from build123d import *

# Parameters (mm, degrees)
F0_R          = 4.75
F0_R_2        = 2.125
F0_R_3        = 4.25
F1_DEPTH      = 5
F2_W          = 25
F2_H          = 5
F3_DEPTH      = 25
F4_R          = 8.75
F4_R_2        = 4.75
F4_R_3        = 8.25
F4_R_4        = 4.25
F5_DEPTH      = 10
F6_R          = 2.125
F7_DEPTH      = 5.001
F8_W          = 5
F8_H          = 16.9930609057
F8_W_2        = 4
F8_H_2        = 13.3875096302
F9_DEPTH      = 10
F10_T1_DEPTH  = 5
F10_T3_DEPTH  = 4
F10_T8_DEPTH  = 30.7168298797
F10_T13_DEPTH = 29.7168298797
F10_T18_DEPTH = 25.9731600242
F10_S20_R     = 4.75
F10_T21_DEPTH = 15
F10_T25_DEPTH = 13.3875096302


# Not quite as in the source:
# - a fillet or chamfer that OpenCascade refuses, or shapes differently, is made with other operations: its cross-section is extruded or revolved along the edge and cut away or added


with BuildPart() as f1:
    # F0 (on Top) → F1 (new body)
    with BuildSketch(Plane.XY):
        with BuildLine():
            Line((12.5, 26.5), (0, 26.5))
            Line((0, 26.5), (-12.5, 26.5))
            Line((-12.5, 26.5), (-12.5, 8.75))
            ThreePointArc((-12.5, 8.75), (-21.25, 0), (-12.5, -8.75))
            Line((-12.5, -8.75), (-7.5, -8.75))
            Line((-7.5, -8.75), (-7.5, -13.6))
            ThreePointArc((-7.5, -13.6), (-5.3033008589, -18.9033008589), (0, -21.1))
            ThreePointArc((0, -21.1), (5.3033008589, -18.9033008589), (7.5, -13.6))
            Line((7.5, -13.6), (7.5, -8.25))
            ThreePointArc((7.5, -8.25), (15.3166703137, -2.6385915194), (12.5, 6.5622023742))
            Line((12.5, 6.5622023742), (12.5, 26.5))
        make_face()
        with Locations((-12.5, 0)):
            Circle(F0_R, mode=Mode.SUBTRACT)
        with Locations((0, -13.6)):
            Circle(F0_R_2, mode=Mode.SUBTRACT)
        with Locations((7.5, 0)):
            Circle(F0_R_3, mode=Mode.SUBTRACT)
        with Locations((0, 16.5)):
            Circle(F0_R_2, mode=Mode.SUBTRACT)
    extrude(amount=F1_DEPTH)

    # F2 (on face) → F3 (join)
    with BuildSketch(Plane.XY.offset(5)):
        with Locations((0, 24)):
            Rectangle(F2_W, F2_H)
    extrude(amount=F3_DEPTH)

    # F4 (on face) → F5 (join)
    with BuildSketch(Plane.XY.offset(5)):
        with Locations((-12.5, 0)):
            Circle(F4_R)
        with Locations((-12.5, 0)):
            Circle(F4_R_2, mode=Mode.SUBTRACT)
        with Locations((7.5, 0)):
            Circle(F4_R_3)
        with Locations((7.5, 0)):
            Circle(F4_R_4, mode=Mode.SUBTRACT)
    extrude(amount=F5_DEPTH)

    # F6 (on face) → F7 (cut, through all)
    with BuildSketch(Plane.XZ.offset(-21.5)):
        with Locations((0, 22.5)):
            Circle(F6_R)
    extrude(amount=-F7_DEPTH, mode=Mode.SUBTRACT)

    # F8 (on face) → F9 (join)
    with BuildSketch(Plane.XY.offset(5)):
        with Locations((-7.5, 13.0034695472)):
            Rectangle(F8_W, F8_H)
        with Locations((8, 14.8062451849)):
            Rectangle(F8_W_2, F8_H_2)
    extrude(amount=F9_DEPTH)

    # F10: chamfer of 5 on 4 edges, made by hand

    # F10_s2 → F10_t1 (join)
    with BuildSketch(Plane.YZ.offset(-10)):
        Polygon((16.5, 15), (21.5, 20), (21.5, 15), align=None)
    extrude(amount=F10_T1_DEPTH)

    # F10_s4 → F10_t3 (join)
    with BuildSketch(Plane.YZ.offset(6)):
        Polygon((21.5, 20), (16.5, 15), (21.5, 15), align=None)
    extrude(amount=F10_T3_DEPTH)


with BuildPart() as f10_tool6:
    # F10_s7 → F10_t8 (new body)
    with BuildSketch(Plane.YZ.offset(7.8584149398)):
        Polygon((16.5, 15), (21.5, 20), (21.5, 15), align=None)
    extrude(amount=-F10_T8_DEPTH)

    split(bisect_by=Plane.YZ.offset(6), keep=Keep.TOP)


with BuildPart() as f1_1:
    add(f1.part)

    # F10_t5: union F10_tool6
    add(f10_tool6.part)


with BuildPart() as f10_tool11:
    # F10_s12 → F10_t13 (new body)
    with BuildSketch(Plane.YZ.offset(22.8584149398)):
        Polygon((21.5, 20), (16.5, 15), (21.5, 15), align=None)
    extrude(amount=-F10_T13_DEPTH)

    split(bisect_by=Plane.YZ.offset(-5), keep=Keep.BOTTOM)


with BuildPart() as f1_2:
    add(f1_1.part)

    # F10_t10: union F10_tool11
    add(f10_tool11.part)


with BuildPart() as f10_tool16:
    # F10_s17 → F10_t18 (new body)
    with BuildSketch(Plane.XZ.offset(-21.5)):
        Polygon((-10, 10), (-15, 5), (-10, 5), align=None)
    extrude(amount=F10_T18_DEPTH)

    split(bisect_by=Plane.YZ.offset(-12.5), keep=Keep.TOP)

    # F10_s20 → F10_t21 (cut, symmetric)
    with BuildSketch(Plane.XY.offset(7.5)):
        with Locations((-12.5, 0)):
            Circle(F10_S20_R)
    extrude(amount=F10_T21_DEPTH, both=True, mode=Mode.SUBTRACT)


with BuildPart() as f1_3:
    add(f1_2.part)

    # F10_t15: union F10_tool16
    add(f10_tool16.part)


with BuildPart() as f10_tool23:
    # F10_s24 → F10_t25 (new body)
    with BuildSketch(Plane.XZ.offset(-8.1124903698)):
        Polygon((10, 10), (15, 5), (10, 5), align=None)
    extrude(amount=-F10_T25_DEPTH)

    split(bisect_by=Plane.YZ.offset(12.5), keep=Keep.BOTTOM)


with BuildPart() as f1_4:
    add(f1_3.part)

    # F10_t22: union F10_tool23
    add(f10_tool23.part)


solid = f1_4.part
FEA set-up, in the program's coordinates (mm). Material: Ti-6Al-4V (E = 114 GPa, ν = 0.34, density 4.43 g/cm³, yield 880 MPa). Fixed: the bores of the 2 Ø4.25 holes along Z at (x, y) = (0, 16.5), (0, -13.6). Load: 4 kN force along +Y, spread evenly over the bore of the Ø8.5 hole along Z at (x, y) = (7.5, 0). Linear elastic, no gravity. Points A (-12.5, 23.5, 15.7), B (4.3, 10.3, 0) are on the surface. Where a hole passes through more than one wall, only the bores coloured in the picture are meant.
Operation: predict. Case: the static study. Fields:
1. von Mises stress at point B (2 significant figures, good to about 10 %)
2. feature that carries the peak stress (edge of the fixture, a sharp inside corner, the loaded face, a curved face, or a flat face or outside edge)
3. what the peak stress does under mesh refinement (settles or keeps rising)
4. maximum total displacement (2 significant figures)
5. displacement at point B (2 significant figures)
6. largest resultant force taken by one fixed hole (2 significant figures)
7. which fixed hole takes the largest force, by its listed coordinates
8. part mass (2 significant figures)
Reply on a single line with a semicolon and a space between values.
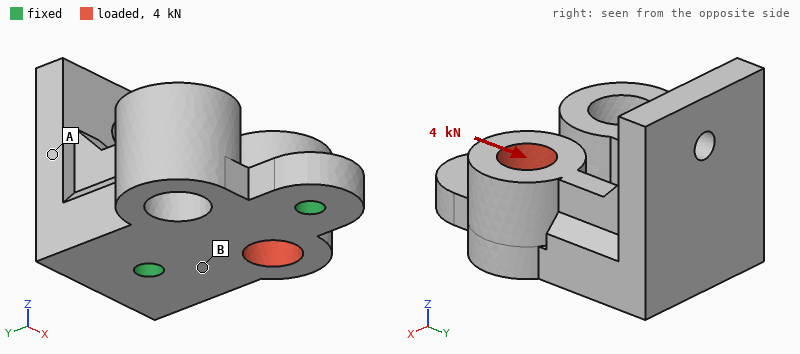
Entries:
23 MPa; edge of the fixture; keeps rising; 15 µm; 2.8 µm; 2.5 kN; (0, 16.5); 58 g
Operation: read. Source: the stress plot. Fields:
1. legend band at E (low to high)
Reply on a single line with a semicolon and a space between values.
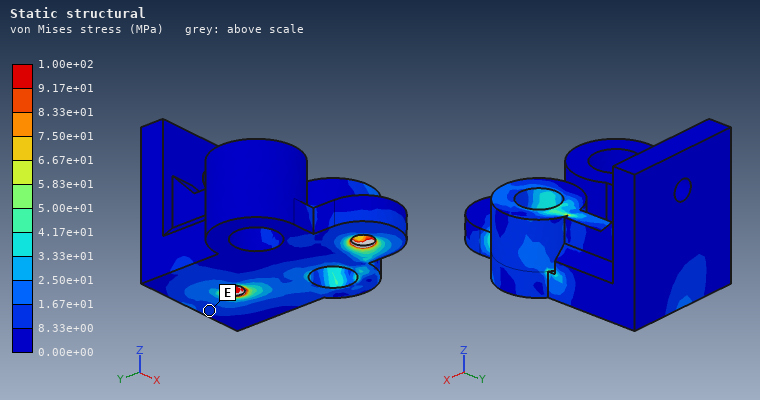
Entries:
8.33e+00 to 1.67e+01 MPa
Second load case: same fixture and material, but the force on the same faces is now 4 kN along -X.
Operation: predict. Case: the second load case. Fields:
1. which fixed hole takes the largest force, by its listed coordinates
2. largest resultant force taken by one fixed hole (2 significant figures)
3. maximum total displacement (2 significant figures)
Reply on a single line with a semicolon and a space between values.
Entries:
(0, -13.6); 2.2 kN; 64 µm
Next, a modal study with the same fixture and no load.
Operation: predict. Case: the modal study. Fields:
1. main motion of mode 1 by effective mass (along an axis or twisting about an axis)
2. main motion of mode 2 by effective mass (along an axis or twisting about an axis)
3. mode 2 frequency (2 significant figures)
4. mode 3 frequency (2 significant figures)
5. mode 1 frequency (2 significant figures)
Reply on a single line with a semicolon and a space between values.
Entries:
along X; along Y; 9300 Hz; 12 kHz; 5600 Hz
